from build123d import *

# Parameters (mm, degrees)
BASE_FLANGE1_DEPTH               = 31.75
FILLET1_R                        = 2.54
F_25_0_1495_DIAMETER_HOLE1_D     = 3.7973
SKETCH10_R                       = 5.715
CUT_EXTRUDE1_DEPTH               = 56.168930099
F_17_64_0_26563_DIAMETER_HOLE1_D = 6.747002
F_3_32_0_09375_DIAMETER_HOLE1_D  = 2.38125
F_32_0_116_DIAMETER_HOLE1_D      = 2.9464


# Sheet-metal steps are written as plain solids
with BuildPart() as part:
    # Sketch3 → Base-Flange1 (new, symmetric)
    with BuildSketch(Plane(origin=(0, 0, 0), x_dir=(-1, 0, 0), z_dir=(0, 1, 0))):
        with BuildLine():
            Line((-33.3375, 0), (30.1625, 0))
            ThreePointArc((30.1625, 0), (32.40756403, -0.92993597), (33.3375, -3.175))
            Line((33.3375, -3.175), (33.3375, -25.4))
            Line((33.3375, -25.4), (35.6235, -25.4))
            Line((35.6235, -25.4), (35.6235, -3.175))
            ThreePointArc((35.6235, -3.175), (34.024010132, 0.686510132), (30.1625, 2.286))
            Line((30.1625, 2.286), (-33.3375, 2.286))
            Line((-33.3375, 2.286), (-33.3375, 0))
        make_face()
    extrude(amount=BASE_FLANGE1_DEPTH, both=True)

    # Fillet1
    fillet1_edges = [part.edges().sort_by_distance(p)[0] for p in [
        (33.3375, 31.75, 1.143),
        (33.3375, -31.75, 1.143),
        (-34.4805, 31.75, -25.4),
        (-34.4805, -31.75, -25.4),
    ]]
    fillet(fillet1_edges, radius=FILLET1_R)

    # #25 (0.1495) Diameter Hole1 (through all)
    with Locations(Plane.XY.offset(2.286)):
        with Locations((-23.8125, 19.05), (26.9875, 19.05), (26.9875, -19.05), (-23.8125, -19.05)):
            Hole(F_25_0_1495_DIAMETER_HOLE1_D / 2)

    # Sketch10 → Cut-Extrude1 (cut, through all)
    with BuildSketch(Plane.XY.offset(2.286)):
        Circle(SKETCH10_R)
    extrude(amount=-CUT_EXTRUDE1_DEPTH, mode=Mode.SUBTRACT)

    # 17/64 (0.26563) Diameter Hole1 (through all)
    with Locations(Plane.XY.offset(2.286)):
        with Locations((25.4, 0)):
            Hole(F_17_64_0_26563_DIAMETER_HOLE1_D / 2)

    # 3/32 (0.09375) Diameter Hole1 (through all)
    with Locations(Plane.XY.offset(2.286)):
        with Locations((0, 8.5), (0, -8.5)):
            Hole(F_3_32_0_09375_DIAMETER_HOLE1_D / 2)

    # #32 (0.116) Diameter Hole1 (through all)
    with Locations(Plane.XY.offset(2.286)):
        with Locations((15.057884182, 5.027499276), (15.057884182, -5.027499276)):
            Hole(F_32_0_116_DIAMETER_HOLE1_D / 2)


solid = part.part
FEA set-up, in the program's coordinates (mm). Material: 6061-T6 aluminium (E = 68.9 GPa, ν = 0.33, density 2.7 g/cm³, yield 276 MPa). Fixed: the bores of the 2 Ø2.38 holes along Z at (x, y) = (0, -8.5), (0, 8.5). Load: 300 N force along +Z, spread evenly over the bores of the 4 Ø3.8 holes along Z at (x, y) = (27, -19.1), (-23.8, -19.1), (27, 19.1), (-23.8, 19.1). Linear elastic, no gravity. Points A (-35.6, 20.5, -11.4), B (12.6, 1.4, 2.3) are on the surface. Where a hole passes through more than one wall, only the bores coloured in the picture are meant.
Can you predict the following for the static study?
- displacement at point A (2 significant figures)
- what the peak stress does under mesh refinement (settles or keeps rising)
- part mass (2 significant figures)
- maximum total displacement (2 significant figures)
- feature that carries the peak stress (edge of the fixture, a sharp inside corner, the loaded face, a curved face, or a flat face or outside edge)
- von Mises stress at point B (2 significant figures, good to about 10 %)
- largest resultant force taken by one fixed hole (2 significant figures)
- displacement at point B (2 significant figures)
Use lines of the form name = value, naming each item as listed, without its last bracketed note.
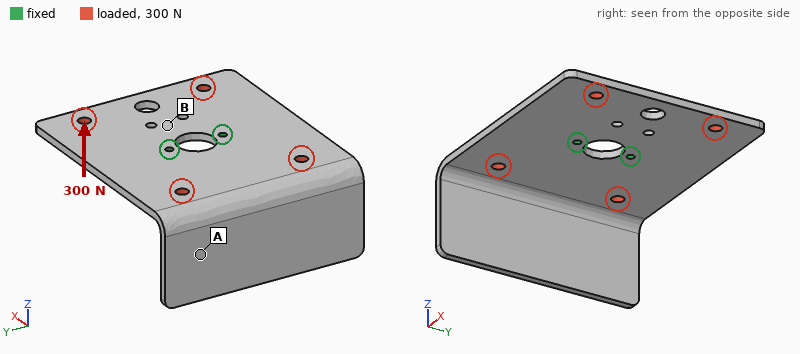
displacement at point A = 0.28 mm
what the peak stress does under mesh refinement = keeps rising
part mass = 35 g
maximum total displacement = 0.36 mm
feature that carries the peak stress = edge of the fixture
von Mises stress at point B = 30 MPa
largest resultant force taken by one fixed hole = 150 N
displacement at point B = 0.072 mm
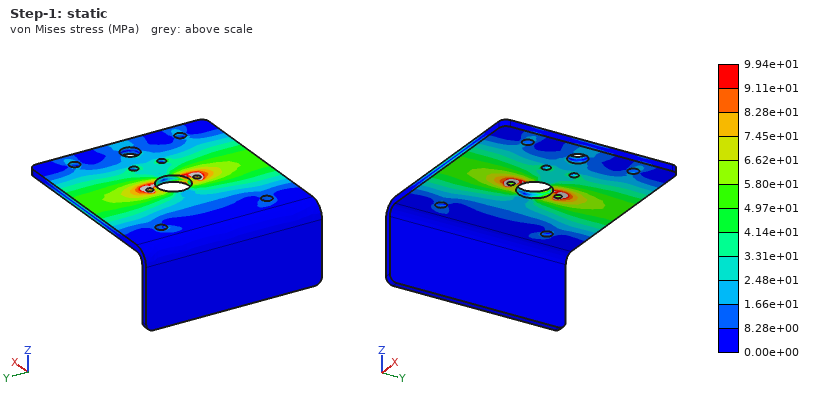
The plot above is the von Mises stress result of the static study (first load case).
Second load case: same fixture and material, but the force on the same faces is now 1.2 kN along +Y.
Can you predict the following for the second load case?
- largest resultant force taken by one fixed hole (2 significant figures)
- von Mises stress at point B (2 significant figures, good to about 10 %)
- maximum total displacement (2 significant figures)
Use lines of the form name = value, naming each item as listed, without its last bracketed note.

largest resultant force taken by one fixed hole = 610 N
von Mises stress at point B = 13 MPa
maximum total displacement = 14 µm
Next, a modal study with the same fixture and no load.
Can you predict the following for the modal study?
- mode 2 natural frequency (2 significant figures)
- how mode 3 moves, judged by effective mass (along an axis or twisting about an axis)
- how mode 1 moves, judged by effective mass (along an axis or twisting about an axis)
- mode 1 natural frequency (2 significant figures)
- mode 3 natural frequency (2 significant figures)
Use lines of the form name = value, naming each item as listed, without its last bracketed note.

mode 2 natural frequency = 960 Hz
how mode 3 moves, judged by effective mass = along Z
how mode 1 moves, judged by effective mass = along Z
mode 1 natural frequency = 560 Hz
mode 3 natural frequency = 1400 Hz
